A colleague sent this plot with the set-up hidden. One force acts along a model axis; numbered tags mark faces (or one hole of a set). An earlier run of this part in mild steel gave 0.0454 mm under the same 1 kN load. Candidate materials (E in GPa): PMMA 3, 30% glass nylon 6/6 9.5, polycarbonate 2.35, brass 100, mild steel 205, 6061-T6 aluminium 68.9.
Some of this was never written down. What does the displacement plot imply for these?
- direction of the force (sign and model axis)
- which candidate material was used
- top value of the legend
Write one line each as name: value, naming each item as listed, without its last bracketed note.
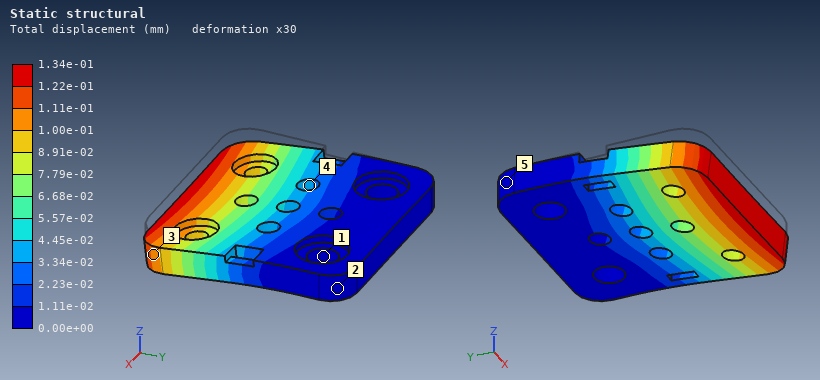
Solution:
direction of the force: -Z
which candidate material was used: 6061-T6 aluminium
top value of the legend: 1.34e-01 mm
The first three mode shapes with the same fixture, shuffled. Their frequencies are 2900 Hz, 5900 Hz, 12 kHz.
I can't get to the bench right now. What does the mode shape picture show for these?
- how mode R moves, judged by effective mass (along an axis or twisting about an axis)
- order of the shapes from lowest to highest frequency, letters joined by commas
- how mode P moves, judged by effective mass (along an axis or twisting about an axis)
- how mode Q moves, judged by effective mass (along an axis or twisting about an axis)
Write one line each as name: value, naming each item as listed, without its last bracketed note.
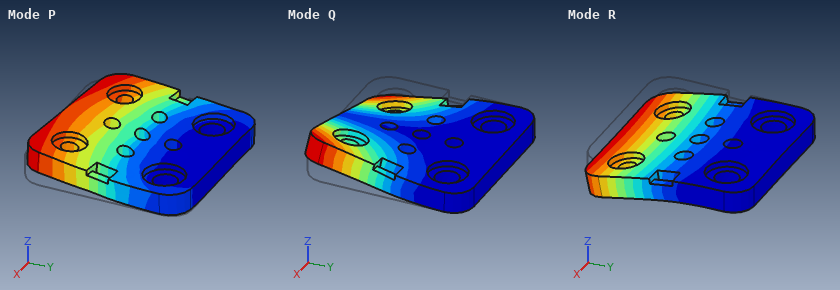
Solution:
how mode R moves, judged by effective mass: along Z
order of the shapes from lowest to highest frequency, letters joined by commas: R, Q, P
how mode P moves, judged by effective mass: along X
how mode Q moves, judged by effective mass: twisting about Y
